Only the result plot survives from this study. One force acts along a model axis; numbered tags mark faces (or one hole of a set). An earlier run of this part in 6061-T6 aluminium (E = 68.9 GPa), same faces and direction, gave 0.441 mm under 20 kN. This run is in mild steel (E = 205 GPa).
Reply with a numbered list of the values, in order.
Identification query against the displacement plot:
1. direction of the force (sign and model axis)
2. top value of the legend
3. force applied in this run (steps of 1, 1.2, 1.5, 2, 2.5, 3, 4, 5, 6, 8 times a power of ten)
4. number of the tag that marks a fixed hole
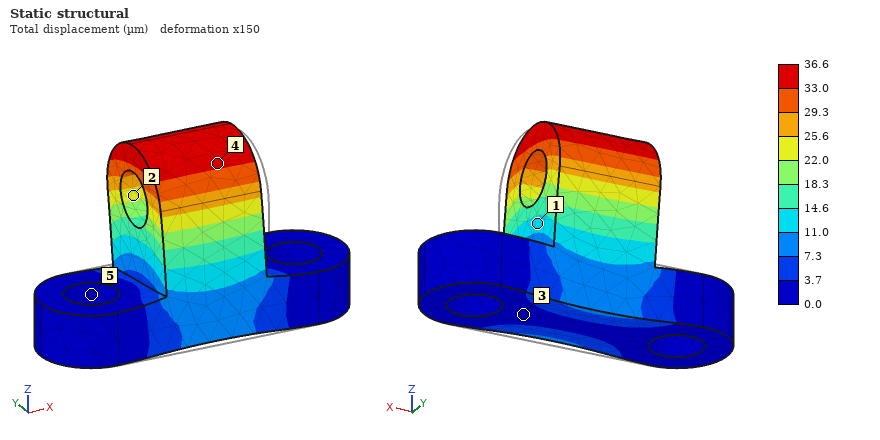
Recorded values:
1. +Y
2. 36.6 µm
3. 5 kN
4. 5
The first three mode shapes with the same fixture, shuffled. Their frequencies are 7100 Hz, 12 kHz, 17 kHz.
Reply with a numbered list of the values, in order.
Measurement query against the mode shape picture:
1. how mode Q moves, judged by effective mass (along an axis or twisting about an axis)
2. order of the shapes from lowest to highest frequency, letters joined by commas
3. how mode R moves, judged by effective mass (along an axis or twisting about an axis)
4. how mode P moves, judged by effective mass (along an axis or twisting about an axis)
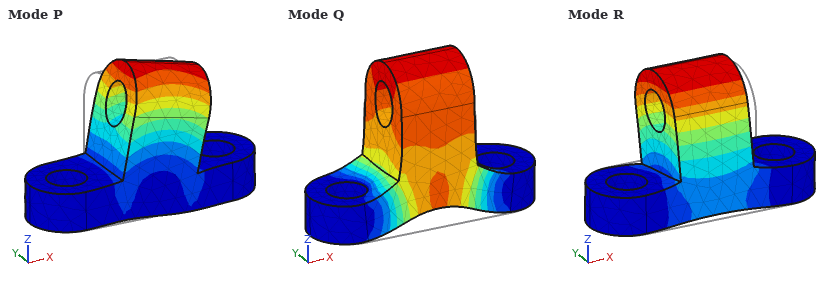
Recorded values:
1. along Z
2. R, P, Q
3. along Y
4. along X
